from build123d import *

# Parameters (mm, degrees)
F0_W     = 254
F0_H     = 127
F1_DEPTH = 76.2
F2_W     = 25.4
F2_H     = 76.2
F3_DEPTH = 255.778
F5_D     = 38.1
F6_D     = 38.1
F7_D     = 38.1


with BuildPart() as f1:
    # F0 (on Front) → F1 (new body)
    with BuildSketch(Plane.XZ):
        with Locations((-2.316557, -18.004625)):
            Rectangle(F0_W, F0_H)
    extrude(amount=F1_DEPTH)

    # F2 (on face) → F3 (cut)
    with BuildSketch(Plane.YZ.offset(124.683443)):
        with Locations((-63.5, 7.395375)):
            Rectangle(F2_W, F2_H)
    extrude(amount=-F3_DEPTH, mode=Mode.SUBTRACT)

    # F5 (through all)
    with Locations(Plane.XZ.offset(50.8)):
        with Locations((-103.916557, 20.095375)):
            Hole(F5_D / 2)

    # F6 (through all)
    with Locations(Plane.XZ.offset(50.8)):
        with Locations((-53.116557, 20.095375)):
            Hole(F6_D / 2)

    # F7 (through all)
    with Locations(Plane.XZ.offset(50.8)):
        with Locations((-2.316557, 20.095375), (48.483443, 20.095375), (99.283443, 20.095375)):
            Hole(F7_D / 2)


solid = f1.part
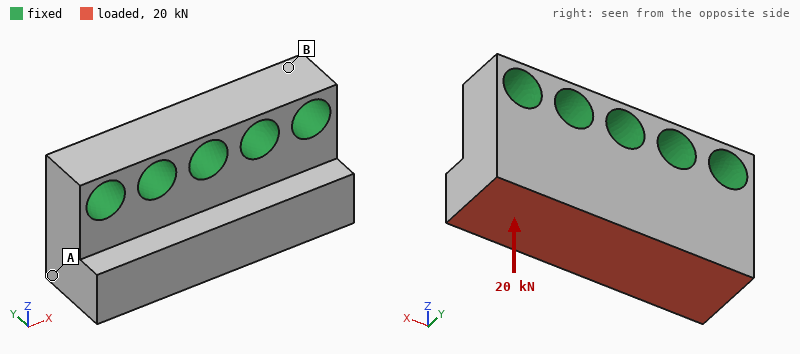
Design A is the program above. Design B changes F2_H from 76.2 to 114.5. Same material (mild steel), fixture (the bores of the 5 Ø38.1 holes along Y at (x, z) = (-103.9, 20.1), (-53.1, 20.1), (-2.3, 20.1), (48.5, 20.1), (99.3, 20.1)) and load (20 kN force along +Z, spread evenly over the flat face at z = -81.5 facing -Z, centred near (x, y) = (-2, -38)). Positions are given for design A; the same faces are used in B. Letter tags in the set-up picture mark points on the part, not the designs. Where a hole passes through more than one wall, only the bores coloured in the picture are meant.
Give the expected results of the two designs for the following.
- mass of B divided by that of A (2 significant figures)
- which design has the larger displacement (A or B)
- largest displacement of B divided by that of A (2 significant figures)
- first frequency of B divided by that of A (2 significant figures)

0.93
B
1.3
1.0
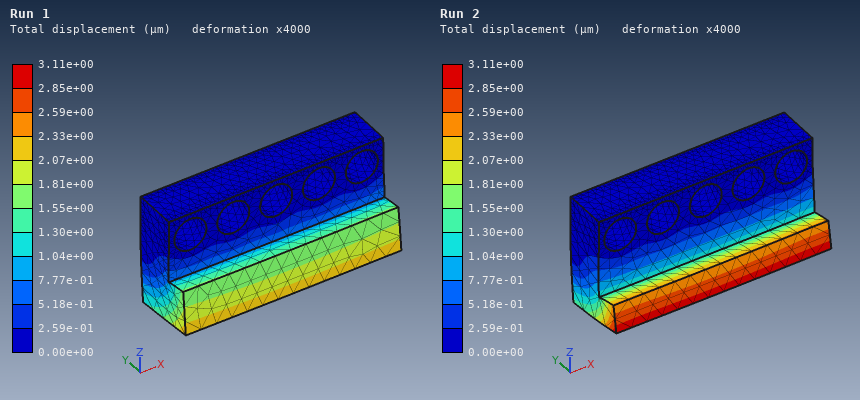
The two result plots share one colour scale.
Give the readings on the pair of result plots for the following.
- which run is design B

Run 2
